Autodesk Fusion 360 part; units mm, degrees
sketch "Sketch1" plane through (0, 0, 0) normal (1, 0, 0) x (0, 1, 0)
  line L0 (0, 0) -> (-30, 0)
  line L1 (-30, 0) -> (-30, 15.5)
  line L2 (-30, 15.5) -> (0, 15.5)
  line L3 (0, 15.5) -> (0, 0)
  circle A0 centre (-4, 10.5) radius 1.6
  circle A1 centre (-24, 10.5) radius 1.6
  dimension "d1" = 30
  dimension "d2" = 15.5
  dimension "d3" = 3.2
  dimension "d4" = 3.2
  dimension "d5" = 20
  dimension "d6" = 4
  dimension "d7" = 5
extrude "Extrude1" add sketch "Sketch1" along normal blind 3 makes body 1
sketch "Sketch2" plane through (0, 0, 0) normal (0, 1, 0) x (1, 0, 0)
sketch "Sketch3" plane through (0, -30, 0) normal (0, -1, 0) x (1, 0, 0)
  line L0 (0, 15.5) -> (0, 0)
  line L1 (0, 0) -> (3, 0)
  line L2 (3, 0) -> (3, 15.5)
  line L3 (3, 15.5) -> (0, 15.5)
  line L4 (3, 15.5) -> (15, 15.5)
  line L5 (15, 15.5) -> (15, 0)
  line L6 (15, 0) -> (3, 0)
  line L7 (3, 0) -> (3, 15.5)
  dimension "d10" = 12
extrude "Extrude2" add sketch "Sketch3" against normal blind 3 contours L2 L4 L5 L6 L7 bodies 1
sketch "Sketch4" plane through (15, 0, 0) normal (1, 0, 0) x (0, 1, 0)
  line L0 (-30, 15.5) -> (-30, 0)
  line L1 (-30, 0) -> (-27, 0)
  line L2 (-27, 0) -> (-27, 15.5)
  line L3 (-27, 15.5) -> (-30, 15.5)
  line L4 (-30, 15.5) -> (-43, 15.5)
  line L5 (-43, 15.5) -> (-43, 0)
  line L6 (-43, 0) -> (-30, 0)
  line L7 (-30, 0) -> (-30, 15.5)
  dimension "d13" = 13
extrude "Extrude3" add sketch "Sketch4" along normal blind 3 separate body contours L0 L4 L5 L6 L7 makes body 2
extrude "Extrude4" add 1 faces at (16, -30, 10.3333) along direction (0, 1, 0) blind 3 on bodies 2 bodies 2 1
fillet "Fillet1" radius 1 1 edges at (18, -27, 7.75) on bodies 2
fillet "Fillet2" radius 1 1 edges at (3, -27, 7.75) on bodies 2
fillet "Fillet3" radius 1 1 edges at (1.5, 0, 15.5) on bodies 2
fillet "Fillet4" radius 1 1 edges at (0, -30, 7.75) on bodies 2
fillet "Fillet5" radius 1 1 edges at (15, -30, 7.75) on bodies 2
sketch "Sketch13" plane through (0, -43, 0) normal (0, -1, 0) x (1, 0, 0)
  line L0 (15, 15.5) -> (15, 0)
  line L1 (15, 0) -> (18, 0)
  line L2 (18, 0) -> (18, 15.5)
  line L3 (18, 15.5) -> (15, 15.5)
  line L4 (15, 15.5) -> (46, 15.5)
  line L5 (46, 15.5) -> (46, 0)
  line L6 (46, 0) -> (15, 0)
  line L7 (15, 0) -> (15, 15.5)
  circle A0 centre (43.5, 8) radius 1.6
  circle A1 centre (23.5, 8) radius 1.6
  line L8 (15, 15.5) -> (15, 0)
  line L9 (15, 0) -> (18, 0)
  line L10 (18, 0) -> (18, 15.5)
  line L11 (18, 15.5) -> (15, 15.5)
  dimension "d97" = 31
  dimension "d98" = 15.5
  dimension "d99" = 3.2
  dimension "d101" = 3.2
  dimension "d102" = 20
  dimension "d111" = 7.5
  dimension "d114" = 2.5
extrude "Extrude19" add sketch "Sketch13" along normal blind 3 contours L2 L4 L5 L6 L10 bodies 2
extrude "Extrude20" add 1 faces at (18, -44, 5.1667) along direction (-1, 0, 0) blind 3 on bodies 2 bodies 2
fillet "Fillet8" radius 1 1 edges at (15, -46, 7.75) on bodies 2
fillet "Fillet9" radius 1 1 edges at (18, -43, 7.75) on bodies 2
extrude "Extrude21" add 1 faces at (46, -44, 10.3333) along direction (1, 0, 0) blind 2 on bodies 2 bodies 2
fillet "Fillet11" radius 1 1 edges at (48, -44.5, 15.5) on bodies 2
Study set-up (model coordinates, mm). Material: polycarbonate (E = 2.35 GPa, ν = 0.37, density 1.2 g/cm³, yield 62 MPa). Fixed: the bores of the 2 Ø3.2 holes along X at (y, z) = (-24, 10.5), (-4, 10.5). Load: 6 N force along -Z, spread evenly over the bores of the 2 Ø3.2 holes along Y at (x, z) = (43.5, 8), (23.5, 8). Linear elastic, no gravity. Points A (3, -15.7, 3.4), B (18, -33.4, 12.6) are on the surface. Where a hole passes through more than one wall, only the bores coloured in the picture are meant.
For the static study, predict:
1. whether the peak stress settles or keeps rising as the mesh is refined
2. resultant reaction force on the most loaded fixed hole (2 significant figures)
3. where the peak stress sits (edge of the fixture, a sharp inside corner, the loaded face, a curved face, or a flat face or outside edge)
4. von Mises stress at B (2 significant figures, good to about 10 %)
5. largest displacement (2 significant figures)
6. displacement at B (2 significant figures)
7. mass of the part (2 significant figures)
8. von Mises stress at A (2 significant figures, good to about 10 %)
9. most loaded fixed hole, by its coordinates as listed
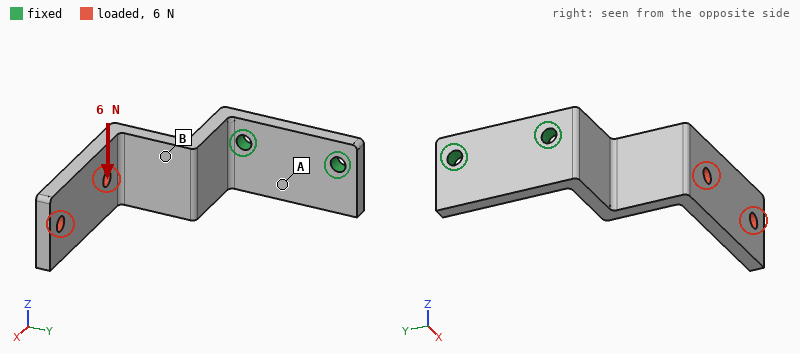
keeps rising
11 N
edge of the fixture
2.8 MPa
0.65 mm
0.12 mm
5.0 g
0.94 MPa
(-24, 10.5)
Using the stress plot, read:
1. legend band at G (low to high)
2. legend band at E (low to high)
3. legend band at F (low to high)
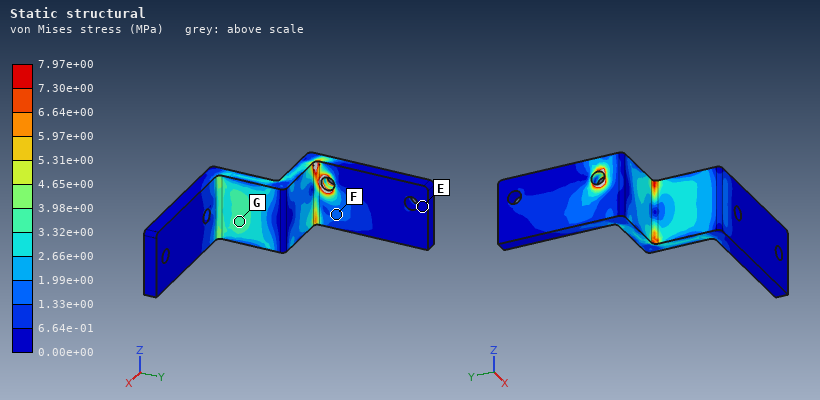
3.32e+00 to 3.98e+00 MPa
0.00e+00 to 6.64e-01 MPa
1.33e+00 to 1.99e+00 MPa
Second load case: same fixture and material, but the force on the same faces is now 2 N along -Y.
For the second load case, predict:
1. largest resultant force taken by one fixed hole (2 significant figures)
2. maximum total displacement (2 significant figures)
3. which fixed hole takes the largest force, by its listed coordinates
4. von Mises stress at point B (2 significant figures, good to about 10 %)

2.2 N
0.75 mm
(-24, 10.5)
1.4 MPa
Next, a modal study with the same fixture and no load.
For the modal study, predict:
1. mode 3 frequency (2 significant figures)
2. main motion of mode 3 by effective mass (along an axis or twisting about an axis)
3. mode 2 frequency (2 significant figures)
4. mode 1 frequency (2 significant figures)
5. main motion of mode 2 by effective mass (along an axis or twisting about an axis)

970 Hz
along X
440 Hz
220 Hz
along Z
